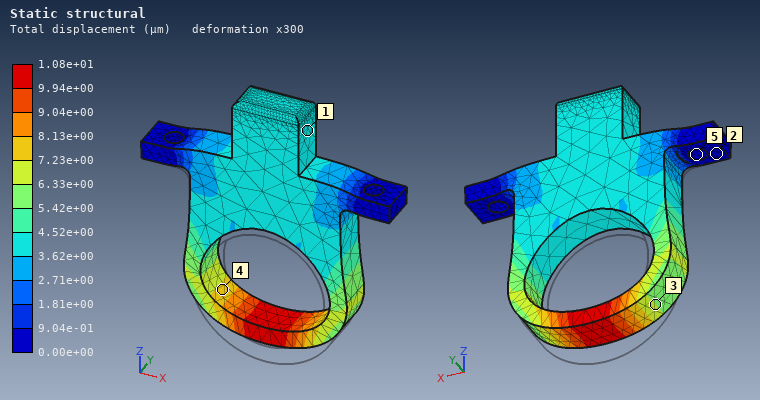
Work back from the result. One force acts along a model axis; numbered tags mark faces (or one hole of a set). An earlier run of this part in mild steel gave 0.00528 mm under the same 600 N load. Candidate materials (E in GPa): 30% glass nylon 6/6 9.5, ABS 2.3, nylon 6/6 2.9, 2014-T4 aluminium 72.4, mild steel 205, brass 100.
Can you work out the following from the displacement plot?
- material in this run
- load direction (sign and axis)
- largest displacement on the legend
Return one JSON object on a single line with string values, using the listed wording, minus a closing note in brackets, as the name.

{"material in this run": "brass", "load direction": "+Z", "largest displacement on the legend": "1.08e+01 µm"}
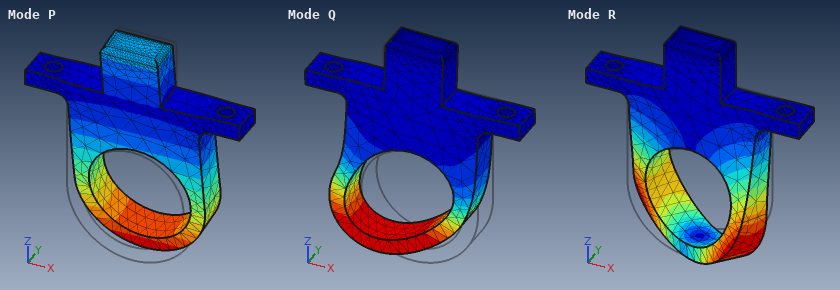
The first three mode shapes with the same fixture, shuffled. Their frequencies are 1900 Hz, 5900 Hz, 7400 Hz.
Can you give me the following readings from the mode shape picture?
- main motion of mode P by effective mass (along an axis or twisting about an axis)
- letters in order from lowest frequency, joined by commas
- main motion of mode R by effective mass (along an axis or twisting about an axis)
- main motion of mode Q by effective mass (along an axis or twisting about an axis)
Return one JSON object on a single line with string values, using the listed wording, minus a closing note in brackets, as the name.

{"main motion of mode P by effective mass": "along Y", "letters in order from lowest frequency, joined by commas": "P, Q, R", "main motion of mode R by effective mass": "twisting about Z", "main motion of mode Q by effective mass": "along X"}
